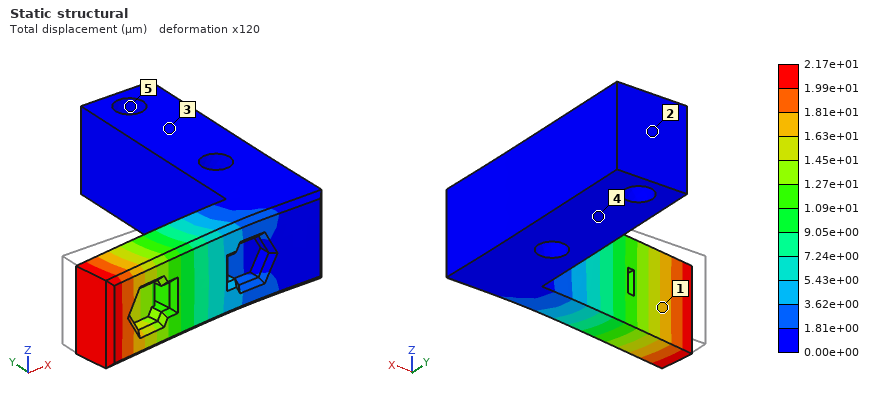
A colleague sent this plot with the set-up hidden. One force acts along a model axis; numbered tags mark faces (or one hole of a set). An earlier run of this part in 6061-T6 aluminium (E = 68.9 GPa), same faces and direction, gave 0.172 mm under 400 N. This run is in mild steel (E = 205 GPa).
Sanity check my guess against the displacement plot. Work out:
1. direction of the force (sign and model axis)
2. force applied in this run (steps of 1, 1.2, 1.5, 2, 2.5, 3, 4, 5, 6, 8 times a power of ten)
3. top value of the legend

-Y
150 N
2.17e+01 µm
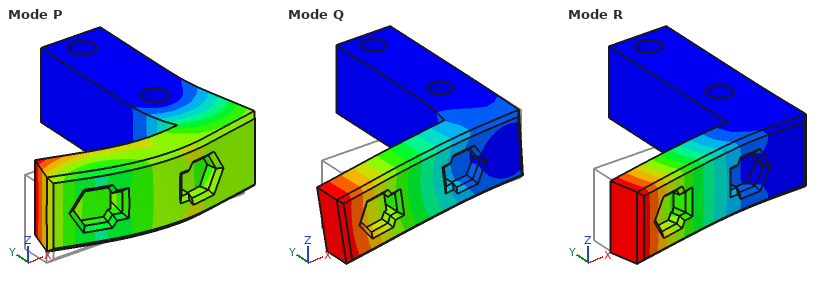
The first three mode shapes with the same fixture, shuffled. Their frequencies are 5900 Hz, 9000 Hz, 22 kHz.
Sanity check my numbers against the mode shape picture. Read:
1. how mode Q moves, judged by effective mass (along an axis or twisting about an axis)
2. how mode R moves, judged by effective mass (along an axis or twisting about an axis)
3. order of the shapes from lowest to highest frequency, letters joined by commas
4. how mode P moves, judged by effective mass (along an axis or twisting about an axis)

along Z
along Y
R, Q, P
along X
